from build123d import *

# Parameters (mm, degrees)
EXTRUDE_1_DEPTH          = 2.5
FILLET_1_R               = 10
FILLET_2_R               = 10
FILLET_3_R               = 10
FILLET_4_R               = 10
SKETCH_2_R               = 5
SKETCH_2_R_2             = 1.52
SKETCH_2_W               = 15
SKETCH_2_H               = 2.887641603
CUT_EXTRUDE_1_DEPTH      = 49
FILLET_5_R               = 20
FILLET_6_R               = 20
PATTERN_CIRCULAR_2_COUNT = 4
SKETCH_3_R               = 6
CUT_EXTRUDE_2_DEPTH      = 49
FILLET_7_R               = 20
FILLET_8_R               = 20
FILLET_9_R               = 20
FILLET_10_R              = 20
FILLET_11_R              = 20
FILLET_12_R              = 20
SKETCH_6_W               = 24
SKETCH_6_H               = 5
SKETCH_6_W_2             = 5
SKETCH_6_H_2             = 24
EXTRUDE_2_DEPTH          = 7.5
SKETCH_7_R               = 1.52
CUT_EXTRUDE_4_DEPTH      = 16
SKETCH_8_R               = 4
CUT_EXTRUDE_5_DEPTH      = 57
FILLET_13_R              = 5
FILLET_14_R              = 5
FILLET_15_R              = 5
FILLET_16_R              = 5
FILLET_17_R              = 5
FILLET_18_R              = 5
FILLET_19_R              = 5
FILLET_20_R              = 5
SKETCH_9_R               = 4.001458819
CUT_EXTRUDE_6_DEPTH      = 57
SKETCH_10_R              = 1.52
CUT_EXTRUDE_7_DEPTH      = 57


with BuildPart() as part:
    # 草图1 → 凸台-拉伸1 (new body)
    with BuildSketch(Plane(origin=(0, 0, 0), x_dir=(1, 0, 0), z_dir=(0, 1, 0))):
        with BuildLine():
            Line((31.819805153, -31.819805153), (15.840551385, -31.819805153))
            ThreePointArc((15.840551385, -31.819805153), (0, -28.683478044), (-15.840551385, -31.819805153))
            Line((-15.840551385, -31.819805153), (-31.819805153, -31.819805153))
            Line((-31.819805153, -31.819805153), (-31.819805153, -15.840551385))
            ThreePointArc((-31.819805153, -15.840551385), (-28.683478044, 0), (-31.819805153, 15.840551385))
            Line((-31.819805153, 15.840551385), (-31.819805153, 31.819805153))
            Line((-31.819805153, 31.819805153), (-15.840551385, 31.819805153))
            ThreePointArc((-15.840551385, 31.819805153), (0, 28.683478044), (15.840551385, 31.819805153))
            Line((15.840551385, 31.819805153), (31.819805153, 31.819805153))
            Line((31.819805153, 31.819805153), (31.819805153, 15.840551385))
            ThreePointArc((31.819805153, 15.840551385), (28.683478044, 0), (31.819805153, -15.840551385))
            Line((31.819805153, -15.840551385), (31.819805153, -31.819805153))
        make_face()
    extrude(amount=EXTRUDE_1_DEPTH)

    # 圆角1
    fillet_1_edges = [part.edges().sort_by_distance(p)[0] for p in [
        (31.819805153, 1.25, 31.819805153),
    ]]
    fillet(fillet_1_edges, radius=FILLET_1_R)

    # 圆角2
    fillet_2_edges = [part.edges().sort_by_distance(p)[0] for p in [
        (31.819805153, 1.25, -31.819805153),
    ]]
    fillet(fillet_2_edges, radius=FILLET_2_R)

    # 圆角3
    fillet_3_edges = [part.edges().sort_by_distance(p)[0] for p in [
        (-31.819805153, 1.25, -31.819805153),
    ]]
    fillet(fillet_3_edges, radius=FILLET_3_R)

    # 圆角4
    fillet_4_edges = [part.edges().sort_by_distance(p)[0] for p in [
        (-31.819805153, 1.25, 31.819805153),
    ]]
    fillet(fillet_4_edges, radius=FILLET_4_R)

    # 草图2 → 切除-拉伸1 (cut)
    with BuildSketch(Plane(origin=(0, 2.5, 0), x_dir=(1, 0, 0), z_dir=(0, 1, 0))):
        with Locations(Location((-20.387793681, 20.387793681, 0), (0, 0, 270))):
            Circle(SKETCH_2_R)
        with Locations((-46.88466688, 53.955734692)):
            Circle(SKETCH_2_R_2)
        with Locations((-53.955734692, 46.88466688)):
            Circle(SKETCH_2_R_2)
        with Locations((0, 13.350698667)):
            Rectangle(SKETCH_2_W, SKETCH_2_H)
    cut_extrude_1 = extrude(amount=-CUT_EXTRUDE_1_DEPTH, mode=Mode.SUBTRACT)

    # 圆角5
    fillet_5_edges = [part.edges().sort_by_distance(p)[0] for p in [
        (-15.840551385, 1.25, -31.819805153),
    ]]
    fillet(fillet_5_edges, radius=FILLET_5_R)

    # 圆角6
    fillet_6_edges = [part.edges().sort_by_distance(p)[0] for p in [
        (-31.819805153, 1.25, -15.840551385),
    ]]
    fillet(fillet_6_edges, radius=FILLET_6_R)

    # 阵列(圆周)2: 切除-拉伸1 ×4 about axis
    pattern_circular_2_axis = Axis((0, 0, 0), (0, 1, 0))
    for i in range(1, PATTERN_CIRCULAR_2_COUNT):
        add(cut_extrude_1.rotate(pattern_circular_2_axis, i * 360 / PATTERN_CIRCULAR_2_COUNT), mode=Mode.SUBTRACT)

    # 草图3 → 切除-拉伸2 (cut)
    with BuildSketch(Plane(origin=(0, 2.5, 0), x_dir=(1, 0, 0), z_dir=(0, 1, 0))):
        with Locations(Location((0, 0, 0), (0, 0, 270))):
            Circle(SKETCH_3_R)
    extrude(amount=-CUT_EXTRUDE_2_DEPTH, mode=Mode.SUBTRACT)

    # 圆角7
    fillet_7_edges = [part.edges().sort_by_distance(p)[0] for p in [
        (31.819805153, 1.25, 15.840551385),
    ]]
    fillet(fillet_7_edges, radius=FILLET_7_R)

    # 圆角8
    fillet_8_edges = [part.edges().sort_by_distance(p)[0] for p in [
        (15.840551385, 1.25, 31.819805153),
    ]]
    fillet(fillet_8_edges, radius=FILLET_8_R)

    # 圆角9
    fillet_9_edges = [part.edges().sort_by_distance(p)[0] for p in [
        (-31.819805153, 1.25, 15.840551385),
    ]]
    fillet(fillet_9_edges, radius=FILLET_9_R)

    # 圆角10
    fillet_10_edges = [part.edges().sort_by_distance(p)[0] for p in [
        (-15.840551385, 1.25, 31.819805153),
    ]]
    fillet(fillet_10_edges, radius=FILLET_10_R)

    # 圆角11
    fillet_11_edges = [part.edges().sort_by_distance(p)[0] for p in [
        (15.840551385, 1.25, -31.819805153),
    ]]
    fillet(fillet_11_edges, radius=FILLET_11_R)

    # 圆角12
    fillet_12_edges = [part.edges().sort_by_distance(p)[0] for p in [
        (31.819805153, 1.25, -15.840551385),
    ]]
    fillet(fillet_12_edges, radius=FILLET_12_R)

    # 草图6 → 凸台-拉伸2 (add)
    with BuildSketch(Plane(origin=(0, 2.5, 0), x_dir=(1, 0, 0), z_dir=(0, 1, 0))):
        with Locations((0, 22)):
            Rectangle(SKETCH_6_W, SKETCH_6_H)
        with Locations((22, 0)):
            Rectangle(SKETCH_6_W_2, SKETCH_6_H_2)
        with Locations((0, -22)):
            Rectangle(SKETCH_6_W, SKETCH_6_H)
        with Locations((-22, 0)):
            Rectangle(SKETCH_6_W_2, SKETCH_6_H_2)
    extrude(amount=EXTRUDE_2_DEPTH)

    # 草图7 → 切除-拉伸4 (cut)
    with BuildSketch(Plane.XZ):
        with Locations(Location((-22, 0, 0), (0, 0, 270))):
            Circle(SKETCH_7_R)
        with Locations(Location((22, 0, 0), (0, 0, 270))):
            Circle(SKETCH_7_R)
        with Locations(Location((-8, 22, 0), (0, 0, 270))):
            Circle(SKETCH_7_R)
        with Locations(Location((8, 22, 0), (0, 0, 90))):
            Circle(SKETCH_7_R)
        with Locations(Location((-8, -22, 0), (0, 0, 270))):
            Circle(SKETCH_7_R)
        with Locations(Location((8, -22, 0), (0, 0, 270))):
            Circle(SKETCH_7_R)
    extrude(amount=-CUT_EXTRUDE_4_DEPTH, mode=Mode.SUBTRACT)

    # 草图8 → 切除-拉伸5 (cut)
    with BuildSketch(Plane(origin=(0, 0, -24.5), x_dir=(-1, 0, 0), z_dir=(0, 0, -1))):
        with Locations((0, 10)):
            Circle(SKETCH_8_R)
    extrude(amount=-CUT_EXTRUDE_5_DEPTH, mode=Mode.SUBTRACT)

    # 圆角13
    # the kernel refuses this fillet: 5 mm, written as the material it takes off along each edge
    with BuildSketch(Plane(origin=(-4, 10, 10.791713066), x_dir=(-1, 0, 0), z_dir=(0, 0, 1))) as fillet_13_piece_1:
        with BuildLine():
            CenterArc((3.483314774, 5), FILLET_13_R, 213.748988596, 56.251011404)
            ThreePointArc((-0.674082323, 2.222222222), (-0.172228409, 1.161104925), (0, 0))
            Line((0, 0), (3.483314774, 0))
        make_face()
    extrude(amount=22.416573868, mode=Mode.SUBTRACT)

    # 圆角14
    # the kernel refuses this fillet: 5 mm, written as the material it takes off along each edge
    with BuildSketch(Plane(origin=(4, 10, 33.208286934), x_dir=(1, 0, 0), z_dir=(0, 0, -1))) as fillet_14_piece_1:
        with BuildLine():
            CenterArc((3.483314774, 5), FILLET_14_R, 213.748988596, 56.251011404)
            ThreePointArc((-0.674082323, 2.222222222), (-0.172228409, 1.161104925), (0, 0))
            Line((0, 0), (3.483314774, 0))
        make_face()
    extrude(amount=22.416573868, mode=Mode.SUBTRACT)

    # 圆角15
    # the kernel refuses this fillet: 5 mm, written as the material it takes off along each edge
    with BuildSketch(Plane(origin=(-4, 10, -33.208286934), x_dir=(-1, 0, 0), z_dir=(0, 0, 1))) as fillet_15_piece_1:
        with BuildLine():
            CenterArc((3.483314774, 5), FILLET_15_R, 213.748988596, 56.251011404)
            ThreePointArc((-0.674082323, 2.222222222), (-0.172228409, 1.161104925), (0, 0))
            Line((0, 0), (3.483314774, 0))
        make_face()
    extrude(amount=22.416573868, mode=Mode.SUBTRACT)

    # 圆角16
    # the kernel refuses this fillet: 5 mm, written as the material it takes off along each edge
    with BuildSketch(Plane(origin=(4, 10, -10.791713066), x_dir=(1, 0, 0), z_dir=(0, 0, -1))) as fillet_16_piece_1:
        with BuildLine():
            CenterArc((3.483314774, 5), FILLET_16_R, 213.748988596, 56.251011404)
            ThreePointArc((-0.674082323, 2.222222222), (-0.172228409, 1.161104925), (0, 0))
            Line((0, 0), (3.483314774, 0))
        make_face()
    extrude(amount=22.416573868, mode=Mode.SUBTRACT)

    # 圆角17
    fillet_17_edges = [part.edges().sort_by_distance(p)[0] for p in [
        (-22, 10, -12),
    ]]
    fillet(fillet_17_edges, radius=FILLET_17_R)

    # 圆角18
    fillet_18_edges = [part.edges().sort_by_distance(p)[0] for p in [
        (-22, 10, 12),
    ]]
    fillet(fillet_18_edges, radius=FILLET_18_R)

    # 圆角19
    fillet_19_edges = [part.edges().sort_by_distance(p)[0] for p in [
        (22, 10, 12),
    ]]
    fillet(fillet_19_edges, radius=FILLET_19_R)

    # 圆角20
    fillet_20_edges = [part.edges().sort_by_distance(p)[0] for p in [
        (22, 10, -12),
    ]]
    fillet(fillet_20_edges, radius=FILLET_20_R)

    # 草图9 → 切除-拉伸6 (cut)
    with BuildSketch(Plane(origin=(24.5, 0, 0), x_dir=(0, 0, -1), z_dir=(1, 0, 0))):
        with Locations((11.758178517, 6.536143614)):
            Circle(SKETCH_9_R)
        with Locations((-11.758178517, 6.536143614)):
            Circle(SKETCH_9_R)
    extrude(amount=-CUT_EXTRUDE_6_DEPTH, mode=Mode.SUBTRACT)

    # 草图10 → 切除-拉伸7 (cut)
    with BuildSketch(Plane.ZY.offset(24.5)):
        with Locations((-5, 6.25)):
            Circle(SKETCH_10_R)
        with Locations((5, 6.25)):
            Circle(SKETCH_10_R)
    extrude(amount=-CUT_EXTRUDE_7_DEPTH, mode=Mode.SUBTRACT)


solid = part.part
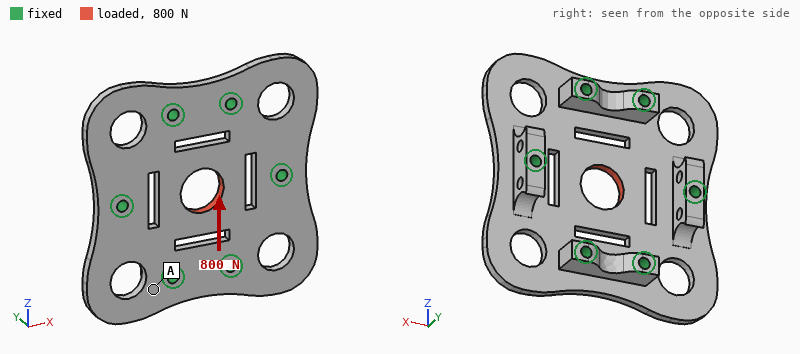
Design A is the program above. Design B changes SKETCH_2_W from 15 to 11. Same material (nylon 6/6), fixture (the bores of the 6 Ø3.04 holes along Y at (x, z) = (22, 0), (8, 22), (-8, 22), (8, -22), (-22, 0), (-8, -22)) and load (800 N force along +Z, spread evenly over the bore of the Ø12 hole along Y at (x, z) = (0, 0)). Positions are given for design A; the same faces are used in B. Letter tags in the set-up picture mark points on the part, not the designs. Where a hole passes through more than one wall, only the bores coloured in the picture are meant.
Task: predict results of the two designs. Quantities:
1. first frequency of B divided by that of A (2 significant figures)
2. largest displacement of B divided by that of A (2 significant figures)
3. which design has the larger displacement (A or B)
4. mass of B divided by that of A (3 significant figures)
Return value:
1.0
0.71
A
1.01
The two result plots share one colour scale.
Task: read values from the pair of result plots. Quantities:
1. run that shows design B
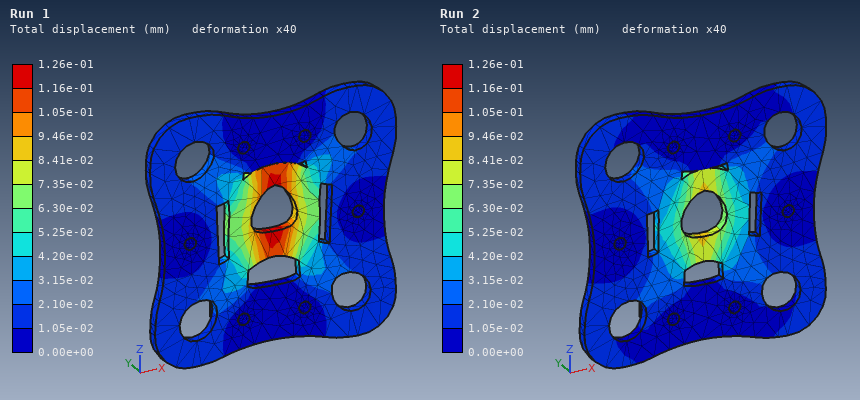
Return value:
Run 2
